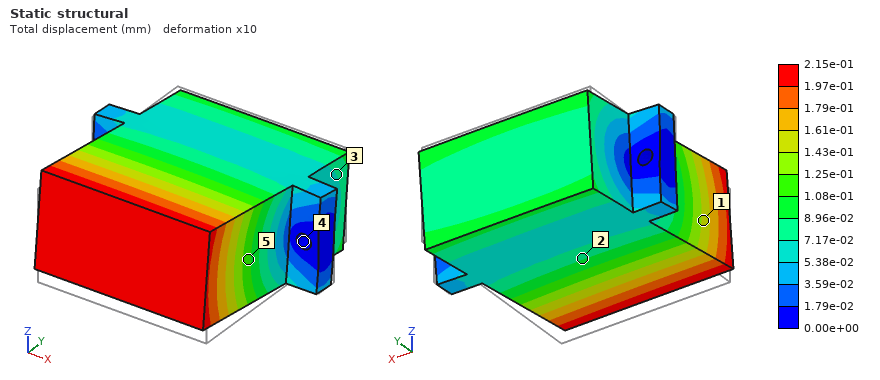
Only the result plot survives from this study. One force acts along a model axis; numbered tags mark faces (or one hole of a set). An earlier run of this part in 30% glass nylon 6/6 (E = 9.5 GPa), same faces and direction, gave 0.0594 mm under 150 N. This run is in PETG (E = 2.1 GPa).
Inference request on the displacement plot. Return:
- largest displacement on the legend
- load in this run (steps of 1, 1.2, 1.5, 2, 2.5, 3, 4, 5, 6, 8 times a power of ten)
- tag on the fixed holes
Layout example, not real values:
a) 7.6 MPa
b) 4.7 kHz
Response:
a) 2.15e-01 mm
b) 120 N
c) 4
